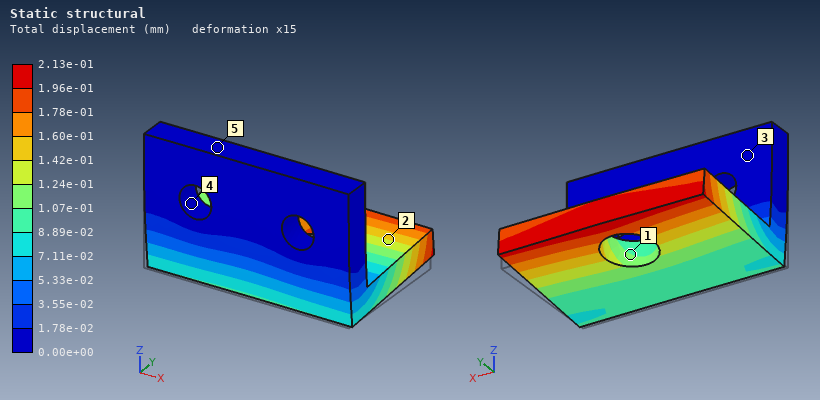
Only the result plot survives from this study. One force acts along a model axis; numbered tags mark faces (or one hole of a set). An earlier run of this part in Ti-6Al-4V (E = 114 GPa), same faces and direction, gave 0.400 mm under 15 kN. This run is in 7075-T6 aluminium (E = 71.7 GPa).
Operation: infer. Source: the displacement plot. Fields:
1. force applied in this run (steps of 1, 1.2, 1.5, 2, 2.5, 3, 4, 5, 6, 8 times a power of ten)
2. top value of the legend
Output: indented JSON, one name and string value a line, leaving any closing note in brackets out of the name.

{
  "force applied in this run": "5 kN",
  "top value of the legend": "2.13e-01 mm"
}
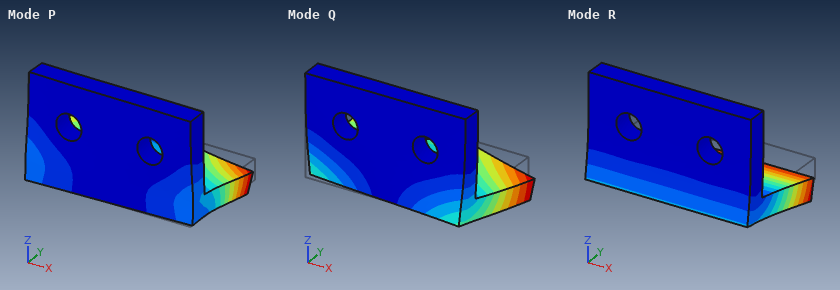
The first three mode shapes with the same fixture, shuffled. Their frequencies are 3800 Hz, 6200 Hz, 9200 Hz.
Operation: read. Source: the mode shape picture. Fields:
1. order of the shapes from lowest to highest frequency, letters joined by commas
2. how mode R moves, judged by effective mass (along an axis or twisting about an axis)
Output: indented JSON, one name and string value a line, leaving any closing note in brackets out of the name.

{
  "order of the shapes from lowest to highest frequency, letters joined by commas": "R, Q, P",
  "how mode R moves, judged by effective mass": "along Z"
}
